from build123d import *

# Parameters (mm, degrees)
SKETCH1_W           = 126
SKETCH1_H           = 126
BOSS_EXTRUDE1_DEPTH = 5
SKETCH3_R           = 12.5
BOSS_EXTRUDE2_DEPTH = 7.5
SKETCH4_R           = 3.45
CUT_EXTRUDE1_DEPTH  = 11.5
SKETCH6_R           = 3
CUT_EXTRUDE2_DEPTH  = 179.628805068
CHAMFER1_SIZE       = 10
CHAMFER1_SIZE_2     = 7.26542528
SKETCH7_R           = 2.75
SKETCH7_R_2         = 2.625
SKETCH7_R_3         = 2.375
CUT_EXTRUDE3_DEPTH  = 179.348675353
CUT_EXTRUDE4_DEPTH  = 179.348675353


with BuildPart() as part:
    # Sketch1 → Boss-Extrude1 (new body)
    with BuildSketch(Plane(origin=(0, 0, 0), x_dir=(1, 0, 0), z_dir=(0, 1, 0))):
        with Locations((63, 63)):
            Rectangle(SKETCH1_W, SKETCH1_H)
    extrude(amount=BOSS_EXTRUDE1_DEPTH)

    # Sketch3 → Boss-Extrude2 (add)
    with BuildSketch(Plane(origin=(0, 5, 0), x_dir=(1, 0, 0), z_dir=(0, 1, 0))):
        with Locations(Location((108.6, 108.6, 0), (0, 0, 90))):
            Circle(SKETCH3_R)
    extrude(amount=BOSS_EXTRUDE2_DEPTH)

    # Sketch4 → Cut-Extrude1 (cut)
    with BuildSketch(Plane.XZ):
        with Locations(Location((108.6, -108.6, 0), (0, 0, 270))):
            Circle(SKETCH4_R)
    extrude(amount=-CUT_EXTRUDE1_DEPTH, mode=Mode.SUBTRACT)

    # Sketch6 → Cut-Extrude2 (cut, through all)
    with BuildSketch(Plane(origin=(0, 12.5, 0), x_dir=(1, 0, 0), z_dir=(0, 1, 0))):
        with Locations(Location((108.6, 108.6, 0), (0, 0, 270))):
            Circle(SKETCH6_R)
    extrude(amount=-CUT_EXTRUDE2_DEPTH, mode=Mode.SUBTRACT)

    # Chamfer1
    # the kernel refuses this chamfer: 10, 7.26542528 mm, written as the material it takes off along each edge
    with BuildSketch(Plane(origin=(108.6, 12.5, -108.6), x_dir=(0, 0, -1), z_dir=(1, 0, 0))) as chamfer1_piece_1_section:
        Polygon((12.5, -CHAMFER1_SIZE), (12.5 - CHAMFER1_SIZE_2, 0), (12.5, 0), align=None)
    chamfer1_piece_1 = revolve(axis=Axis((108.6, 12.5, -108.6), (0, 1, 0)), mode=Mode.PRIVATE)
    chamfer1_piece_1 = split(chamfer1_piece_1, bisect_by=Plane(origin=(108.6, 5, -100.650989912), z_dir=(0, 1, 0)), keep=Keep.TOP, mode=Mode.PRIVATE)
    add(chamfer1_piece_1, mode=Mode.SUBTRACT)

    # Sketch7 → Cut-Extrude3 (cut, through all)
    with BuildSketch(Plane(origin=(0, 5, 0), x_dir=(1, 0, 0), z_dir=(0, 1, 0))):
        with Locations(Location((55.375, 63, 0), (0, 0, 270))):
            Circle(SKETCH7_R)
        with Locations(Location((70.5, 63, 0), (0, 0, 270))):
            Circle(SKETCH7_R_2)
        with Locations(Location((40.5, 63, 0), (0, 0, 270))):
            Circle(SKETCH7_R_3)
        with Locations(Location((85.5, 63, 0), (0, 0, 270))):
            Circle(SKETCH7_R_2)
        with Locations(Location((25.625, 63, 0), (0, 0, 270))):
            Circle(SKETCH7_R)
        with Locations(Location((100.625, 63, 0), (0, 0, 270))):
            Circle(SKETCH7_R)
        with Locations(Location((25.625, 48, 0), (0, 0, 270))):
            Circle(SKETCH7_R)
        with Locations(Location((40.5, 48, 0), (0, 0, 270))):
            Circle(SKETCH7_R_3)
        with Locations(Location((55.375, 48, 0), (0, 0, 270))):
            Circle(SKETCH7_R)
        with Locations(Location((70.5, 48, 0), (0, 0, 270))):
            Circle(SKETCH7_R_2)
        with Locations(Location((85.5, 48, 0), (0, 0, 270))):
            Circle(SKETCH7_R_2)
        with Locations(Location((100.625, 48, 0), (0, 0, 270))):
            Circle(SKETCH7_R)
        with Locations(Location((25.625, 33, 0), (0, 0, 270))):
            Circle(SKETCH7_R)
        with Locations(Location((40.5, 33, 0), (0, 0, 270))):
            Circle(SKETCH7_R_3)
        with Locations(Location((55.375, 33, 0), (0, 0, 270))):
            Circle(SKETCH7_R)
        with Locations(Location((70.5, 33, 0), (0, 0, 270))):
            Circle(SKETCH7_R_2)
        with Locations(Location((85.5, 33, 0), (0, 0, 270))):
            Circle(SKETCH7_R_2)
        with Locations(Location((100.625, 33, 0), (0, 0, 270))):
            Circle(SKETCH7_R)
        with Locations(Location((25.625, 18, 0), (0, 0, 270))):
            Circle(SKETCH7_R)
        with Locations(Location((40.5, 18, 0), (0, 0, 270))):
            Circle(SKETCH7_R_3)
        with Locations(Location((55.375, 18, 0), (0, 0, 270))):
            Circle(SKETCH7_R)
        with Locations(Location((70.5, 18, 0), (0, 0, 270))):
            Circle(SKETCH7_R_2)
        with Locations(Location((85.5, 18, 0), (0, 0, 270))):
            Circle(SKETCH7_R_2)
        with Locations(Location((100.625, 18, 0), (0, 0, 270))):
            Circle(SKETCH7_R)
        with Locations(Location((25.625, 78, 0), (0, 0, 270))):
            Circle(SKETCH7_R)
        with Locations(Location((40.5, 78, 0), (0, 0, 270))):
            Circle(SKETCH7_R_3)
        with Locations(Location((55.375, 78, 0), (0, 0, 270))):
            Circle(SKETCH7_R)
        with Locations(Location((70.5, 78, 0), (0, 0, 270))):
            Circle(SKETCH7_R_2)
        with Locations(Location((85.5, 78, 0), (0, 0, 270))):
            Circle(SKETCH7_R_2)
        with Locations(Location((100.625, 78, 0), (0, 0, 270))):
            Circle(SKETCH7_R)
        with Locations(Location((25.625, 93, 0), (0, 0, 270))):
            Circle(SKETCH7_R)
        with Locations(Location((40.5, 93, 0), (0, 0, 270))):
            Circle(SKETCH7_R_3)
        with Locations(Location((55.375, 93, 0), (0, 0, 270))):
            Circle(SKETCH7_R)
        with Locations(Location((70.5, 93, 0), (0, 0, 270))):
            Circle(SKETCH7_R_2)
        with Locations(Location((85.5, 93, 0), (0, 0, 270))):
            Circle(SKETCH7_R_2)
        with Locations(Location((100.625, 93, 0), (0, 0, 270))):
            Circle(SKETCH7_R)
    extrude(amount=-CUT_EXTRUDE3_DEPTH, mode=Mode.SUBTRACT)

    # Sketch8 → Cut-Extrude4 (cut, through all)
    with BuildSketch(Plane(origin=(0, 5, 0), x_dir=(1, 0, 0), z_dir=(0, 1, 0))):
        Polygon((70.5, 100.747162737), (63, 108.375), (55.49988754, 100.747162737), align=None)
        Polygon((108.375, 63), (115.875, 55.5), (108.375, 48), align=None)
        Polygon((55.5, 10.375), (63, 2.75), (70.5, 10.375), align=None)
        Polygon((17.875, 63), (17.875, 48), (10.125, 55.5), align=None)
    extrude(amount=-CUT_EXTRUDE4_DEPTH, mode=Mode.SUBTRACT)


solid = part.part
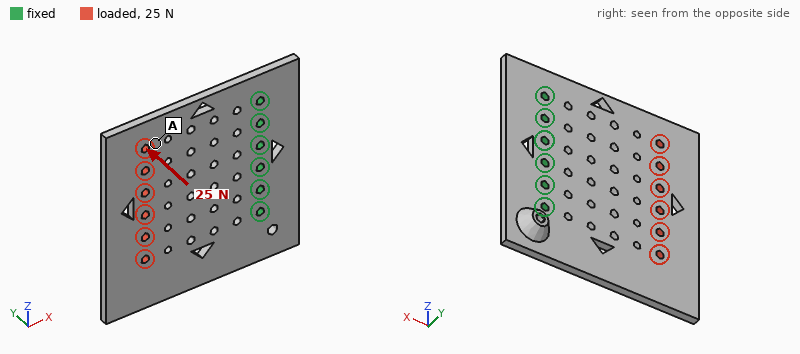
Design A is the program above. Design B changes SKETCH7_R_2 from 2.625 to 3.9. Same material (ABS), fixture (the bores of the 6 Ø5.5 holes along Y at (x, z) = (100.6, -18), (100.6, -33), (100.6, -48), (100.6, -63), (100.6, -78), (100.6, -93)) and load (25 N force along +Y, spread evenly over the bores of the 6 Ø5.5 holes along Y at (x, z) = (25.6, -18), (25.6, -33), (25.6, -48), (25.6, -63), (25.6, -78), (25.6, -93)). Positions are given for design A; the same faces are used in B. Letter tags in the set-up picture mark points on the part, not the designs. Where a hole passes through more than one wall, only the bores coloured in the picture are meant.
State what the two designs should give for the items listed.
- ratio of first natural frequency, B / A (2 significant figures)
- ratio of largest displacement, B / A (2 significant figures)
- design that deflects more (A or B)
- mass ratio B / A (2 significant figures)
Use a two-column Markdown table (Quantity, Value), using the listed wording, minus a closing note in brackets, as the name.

| Quantity | Value |
|---|---|
| ratio of first natural frequency, B / A | 0.95 |
| ratio of largest displacement, B / A | 1.1 |
| design that deflects more | B |
| mass ratio B / A | 0.98 |
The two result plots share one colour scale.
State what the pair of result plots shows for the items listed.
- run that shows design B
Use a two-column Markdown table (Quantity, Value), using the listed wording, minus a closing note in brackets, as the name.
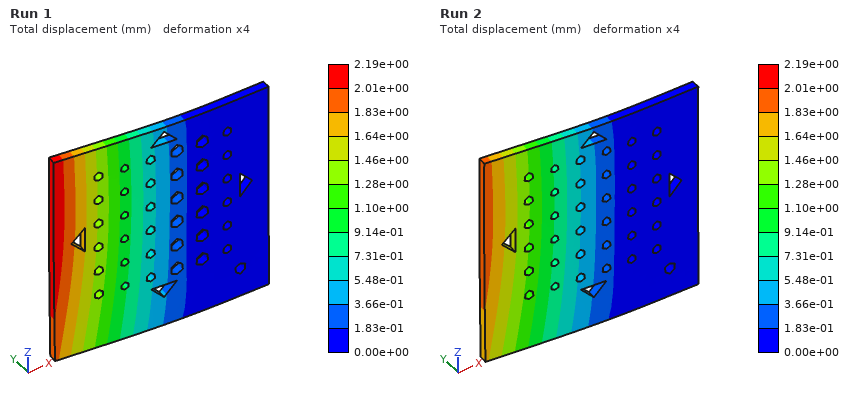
| Quantity | Value |
|---|---|
| run that shows design B | Run 1 |
